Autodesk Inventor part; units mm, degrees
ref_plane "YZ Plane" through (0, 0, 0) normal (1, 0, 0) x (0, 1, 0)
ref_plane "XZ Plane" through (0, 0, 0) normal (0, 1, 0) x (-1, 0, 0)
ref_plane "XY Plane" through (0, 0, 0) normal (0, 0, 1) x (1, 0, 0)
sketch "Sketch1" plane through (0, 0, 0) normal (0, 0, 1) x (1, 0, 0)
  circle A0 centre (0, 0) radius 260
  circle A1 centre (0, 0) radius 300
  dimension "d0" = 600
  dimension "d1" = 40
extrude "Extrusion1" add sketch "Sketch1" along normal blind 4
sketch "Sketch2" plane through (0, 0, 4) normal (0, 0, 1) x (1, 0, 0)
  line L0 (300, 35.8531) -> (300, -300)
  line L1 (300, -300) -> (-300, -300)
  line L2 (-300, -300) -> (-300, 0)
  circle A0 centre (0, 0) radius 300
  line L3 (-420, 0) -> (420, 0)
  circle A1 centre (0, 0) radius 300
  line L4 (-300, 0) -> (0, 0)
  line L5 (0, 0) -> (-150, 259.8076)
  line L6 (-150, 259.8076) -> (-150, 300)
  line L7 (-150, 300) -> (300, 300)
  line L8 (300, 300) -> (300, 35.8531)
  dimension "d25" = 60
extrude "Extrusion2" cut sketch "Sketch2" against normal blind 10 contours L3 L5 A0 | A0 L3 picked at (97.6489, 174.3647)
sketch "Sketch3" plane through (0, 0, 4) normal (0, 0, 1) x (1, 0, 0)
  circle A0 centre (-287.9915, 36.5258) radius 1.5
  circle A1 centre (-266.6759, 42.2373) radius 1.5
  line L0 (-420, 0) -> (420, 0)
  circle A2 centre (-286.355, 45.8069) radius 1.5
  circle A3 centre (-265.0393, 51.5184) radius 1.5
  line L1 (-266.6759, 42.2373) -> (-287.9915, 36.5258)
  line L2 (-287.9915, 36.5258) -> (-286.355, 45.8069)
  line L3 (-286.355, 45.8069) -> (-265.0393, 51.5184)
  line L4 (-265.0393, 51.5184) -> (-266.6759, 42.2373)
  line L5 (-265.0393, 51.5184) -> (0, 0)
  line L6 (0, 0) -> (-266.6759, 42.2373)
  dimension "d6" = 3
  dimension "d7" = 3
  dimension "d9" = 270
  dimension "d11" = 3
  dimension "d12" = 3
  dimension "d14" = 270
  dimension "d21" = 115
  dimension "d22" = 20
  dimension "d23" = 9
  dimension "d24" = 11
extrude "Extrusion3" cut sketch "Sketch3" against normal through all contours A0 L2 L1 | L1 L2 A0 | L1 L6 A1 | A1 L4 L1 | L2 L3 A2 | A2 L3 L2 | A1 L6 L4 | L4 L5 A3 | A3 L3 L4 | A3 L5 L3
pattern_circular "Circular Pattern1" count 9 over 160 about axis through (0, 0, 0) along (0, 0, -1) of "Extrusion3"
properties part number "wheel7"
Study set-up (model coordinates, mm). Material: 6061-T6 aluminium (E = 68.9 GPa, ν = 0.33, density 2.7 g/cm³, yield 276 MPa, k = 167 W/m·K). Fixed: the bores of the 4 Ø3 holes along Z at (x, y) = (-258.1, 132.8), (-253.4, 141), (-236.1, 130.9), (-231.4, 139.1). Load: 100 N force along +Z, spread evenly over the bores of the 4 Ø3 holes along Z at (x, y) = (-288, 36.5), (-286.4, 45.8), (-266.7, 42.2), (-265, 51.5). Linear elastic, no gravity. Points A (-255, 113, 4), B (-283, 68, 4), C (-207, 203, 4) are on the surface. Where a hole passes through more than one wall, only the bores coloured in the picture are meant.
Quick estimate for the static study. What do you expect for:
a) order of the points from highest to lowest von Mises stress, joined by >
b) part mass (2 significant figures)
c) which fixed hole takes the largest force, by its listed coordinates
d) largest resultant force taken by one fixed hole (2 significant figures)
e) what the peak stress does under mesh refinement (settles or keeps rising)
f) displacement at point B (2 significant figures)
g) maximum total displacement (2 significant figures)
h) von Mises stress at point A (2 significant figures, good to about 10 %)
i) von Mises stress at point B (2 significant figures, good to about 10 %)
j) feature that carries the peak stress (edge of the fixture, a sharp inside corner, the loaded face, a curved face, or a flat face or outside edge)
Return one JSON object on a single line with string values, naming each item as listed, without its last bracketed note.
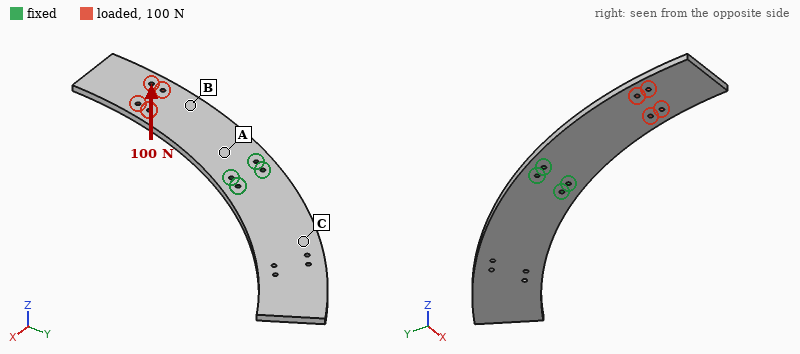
{"order of the points from highest to lowest von Mises stress, joined by >": "A > B > C", "part mass": "130 g", "which fixed hole takes the largest force, by its listed coordinates": "(-258.1, 132.8)", "largest resultant force taken by one fixed hole": "350 N", "what the peak stress does under mesh refinement": "keeps rising", "displacement at point B": "1.1 mm", "maximum total displacement": "3.1 mm", "von Mises stress at point A": "62 MPa", "von Mises stress at point B": "21 MPa", "feature that carries the peak stress": "edge of the fixture"}
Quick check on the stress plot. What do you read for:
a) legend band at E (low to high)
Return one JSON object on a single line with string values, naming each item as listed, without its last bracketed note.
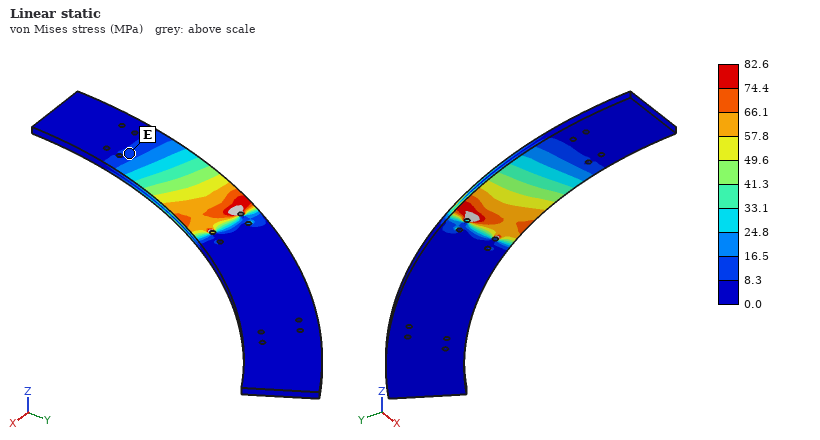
{"legend band at E": "8.3 to 16.5 MPa"}
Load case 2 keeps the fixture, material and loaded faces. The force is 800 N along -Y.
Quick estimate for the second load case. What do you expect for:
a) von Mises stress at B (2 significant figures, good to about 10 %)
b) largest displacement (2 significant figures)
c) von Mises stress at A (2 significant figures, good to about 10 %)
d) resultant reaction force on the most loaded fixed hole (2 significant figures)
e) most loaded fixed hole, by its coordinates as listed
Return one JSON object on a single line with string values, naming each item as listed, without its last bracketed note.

{"von Mises stress at B": "7.0 MPa", "largest displacement": "91 µm", "von Mises stress at A": "7.3 MPa", "resultant reaction force on the most loaded fixed hole": "1.0 kN", "most loaded fixed hole, by its coordinates as listed": "(-258.1, 132.8)"}
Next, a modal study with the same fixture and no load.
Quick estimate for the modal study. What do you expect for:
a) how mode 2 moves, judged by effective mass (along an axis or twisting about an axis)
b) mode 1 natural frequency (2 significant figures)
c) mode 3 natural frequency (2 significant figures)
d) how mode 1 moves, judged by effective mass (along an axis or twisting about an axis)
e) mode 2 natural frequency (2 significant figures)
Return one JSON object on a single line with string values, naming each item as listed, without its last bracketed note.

{"how mode 2 moves, judged by effective mass": "along Z", "mode 1 natural frequency": "160 Hz", "mode 3 natural frequency": "870 Hz", "how mode 1 moves, judged by effective mass": "along Z", "mode 2 natural frequency": "180 Hz"}
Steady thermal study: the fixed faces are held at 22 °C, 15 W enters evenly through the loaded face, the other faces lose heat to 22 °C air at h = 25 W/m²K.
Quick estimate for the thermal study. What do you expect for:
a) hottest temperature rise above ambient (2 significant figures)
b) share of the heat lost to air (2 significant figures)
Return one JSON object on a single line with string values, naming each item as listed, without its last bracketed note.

{"hottest temperature rise above ambient": "35 K", "share of the heat lost to air": "43 %"}
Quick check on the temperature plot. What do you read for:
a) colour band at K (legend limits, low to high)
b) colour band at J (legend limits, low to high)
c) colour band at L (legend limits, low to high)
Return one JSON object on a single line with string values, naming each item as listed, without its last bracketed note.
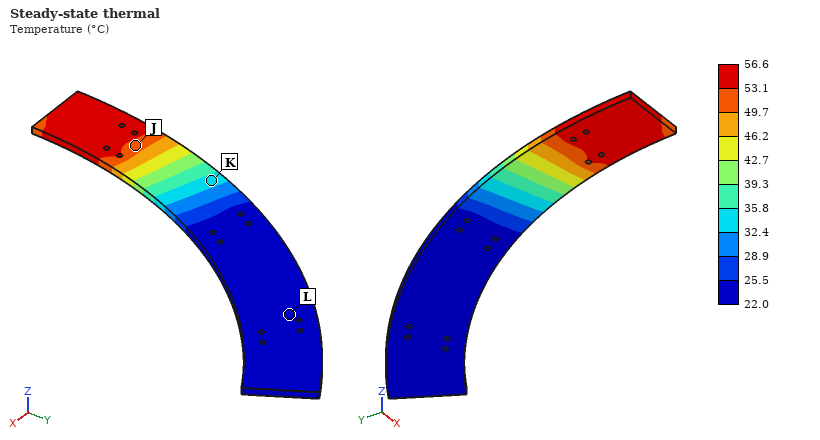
{"colour band at K": "32.4 to 35.8 °C", "colour band at J": "49.7 to 53.1 °C", "colour band at L": "22.0 to 25.5 °C"}
